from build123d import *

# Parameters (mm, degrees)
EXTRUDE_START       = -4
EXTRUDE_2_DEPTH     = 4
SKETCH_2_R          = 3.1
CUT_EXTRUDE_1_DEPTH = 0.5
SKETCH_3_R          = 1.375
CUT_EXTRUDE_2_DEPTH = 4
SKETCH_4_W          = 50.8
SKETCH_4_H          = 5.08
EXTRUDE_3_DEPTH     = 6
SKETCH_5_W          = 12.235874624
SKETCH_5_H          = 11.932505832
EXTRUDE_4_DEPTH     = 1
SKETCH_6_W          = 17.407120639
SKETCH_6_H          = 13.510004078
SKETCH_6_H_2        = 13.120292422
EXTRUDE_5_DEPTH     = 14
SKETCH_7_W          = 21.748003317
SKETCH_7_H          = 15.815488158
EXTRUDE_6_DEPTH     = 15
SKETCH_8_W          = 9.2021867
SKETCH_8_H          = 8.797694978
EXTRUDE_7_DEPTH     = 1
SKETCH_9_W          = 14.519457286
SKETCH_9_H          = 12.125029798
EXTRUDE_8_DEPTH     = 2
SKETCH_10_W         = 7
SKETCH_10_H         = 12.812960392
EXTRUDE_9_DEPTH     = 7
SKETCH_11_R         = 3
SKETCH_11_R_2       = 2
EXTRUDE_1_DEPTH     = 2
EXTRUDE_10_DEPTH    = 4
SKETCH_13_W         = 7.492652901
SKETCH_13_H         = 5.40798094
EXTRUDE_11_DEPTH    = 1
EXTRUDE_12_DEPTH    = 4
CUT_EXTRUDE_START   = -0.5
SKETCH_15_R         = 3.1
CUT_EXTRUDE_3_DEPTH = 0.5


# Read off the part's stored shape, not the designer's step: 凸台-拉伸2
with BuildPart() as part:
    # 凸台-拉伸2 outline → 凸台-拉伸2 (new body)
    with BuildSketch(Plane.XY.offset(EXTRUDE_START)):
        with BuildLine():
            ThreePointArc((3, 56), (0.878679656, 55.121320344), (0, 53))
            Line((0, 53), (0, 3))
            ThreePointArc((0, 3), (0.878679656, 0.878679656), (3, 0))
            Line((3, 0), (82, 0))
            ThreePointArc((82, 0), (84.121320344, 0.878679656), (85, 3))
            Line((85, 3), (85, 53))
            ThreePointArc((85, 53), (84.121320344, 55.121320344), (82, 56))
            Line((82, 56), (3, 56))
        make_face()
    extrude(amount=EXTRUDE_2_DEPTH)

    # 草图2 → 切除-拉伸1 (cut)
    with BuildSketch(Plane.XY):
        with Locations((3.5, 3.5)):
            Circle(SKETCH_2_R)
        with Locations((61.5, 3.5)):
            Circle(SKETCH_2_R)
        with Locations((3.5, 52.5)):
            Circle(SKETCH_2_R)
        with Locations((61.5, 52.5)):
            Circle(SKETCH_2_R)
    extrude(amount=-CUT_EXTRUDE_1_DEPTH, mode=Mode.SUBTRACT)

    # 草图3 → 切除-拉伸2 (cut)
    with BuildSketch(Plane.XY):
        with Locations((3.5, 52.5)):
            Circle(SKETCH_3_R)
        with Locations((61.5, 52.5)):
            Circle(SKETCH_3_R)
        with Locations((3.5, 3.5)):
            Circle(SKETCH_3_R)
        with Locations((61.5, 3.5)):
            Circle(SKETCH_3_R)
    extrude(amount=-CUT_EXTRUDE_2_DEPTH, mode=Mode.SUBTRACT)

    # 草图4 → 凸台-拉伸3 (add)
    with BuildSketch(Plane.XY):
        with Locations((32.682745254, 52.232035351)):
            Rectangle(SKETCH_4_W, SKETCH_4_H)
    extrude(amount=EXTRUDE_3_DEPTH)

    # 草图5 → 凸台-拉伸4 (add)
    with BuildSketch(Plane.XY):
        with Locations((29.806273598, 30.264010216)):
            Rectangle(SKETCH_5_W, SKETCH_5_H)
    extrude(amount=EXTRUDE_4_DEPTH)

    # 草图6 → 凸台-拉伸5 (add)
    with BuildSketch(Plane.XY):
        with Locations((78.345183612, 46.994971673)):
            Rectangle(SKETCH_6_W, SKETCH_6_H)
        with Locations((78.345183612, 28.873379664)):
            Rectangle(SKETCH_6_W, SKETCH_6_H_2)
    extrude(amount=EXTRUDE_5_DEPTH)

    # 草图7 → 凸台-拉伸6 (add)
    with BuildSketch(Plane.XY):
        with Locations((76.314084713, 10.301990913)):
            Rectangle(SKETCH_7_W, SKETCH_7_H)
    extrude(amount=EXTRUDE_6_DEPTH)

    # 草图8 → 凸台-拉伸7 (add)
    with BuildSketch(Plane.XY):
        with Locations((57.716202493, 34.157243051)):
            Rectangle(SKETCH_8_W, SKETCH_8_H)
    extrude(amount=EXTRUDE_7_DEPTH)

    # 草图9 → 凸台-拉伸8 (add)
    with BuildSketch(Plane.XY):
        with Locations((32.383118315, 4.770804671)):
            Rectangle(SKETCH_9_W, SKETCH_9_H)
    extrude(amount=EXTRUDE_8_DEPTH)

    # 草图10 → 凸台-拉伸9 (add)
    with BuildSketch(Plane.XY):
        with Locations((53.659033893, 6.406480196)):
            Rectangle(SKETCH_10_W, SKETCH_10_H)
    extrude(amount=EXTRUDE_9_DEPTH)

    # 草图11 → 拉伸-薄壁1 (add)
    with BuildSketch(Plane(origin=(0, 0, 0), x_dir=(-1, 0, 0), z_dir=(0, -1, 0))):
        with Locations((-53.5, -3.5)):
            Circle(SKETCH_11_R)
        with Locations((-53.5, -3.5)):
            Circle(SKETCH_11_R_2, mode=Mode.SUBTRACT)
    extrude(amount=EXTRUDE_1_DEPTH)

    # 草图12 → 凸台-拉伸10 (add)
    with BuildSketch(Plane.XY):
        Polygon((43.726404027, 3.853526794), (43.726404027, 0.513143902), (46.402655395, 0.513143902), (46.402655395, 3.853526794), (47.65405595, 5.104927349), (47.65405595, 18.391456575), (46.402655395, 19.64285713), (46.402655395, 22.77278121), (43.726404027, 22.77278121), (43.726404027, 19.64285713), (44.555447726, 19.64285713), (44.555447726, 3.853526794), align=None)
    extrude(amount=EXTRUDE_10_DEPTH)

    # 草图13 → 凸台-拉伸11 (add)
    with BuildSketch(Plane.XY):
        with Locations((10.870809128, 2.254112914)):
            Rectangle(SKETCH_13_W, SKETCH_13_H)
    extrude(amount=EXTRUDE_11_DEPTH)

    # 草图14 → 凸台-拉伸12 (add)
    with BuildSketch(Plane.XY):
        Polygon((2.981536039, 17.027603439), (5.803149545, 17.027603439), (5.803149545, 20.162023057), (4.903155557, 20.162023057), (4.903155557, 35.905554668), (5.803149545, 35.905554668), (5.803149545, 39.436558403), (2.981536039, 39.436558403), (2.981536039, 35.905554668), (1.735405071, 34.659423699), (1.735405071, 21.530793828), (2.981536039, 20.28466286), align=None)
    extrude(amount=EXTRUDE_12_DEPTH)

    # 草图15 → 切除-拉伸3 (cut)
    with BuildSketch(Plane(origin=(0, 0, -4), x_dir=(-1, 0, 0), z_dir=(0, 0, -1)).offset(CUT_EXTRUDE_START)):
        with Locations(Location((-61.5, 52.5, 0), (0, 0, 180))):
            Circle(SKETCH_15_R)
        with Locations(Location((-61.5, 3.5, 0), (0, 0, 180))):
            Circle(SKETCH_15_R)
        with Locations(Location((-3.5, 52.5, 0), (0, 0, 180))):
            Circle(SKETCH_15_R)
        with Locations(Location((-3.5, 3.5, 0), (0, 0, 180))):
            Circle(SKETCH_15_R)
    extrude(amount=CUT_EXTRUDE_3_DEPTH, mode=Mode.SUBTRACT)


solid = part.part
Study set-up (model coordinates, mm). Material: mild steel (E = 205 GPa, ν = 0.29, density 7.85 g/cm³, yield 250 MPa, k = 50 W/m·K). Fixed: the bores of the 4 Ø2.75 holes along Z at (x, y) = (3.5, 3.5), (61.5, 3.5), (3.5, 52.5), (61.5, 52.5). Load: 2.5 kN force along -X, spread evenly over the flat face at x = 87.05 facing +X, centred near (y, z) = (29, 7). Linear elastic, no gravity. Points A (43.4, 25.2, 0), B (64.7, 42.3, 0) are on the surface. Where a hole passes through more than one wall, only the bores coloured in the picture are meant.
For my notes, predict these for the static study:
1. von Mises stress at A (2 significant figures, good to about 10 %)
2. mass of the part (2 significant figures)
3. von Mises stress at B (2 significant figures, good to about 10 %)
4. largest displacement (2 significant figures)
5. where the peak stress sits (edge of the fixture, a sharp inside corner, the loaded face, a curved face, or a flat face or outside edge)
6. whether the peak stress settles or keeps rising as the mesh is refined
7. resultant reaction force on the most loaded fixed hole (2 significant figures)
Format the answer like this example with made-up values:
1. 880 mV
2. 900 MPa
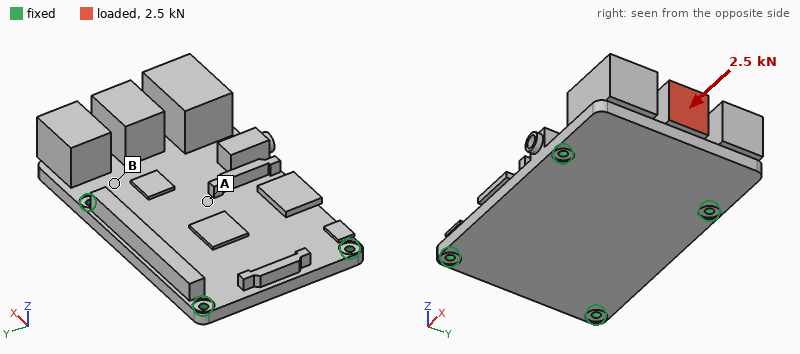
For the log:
1. 35 MPa
2. 270 g
3. 130 MPa
4. 0.16 mm
5. edge of the fixture
6. keeps rising
7. 880 N
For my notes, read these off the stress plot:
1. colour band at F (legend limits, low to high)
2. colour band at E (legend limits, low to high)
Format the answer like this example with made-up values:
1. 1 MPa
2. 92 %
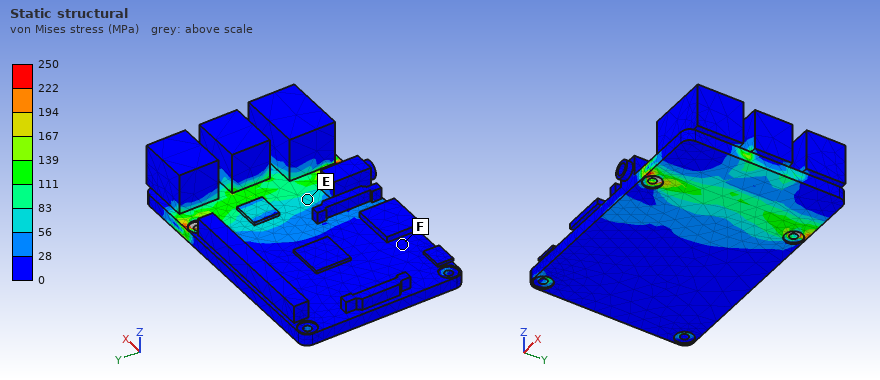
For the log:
1. 0 to 28 MPa
2. 56 to 83 MPa
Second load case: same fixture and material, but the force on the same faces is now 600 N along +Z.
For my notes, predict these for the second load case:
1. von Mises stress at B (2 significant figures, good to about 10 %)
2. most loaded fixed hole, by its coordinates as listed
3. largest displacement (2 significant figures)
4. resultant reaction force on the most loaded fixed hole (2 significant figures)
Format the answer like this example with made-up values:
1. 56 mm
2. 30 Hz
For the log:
1. 75 MPa
2. (61.5, 52.5)
3. 0.11 mm
4. 420 N
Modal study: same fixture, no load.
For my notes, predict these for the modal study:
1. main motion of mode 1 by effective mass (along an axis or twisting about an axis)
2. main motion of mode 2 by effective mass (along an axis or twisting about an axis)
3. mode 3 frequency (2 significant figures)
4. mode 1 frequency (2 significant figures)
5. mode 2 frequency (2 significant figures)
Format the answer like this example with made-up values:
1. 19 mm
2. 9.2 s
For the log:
1. along Z
2. along Z
3. 4500 Hz
4. 1700 Hz
5. 4100 Hz
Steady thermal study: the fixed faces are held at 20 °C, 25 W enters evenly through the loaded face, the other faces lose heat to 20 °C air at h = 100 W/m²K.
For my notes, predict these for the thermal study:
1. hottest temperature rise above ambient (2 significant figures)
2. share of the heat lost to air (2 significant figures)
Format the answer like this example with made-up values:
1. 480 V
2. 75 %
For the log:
1. 68 K
2. 64 %
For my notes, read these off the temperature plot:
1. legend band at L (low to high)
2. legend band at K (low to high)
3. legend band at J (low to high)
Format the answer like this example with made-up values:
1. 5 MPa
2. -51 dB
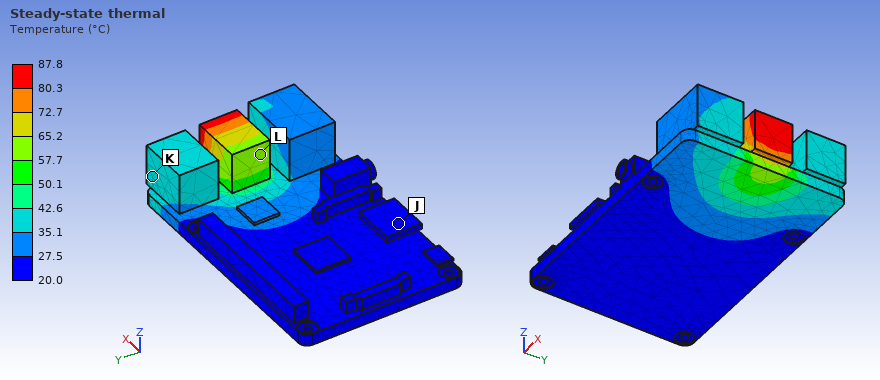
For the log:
1. 57.7 to 65.2 °C
2. 35.1 to 42.6 °C
3. 20.0 to 27.5 °C
